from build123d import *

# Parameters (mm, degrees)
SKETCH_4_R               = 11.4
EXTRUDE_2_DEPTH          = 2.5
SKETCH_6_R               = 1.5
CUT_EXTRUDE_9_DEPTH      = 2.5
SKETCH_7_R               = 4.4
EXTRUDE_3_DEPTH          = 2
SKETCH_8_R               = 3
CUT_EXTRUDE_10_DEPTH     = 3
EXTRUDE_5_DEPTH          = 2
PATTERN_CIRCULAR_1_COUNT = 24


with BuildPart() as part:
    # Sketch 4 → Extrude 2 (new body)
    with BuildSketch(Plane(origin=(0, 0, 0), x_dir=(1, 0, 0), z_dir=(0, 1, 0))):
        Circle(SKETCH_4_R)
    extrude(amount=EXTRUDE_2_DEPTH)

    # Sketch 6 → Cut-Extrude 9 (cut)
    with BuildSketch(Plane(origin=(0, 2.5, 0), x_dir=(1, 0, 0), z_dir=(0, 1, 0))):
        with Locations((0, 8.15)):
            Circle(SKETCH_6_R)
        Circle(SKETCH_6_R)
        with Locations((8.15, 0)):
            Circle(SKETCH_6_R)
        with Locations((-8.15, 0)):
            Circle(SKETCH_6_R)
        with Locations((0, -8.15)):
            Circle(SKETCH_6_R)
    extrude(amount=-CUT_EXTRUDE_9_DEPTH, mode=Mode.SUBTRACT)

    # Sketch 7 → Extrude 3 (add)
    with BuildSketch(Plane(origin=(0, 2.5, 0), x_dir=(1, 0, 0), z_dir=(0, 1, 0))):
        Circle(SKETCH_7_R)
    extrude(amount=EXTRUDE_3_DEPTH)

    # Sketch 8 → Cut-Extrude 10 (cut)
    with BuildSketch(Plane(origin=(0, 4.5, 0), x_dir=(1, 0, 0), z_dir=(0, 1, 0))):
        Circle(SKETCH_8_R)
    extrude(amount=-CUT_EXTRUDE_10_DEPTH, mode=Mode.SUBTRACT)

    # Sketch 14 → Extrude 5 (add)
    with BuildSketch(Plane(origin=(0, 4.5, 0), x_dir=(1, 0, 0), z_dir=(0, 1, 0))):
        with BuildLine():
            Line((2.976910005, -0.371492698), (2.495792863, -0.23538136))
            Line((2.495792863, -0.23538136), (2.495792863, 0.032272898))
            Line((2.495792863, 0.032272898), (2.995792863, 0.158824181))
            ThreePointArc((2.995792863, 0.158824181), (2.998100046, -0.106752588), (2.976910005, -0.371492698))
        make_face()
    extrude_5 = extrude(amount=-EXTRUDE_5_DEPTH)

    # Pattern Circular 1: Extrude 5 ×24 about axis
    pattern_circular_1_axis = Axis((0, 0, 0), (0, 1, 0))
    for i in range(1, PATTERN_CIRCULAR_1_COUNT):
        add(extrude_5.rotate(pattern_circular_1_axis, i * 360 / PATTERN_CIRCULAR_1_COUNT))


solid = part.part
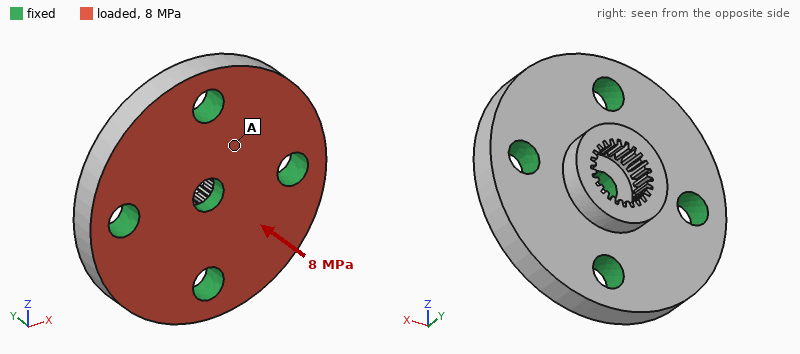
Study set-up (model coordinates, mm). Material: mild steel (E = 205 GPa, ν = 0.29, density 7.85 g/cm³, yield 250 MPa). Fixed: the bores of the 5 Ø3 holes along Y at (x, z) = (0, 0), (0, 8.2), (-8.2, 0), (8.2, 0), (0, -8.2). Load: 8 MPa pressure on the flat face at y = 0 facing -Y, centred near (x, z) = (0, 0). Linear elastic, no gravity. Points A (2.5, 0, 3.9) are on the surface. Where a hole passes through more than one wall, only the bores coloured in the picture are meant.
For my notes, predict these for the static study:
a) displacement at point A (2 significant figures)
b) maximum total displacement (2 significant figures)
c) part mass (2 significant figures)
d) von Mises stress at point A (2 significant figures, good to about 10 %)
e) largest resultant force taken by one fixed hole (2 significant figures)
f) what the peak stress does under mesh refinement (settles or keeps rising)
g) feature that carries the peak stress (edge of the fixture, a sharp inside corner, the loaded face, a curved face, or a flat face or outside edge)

0.82 µm
3.8 µm
7.7 g
22 MPa
660 N
keeps rising
edge of the fixture
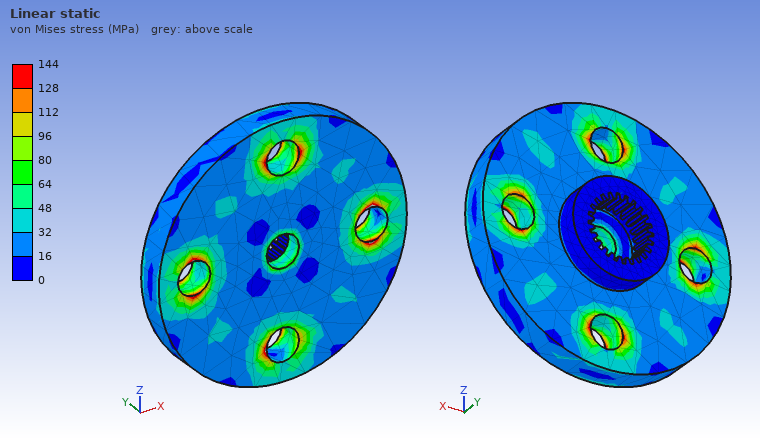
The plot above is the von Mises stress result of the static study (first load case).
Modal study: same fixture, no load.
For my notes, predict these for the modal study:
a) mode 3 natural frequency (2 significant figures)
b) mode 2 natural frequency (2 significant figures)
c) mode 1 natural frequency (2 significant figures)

68 kHz
68 kHz
67 kHz
